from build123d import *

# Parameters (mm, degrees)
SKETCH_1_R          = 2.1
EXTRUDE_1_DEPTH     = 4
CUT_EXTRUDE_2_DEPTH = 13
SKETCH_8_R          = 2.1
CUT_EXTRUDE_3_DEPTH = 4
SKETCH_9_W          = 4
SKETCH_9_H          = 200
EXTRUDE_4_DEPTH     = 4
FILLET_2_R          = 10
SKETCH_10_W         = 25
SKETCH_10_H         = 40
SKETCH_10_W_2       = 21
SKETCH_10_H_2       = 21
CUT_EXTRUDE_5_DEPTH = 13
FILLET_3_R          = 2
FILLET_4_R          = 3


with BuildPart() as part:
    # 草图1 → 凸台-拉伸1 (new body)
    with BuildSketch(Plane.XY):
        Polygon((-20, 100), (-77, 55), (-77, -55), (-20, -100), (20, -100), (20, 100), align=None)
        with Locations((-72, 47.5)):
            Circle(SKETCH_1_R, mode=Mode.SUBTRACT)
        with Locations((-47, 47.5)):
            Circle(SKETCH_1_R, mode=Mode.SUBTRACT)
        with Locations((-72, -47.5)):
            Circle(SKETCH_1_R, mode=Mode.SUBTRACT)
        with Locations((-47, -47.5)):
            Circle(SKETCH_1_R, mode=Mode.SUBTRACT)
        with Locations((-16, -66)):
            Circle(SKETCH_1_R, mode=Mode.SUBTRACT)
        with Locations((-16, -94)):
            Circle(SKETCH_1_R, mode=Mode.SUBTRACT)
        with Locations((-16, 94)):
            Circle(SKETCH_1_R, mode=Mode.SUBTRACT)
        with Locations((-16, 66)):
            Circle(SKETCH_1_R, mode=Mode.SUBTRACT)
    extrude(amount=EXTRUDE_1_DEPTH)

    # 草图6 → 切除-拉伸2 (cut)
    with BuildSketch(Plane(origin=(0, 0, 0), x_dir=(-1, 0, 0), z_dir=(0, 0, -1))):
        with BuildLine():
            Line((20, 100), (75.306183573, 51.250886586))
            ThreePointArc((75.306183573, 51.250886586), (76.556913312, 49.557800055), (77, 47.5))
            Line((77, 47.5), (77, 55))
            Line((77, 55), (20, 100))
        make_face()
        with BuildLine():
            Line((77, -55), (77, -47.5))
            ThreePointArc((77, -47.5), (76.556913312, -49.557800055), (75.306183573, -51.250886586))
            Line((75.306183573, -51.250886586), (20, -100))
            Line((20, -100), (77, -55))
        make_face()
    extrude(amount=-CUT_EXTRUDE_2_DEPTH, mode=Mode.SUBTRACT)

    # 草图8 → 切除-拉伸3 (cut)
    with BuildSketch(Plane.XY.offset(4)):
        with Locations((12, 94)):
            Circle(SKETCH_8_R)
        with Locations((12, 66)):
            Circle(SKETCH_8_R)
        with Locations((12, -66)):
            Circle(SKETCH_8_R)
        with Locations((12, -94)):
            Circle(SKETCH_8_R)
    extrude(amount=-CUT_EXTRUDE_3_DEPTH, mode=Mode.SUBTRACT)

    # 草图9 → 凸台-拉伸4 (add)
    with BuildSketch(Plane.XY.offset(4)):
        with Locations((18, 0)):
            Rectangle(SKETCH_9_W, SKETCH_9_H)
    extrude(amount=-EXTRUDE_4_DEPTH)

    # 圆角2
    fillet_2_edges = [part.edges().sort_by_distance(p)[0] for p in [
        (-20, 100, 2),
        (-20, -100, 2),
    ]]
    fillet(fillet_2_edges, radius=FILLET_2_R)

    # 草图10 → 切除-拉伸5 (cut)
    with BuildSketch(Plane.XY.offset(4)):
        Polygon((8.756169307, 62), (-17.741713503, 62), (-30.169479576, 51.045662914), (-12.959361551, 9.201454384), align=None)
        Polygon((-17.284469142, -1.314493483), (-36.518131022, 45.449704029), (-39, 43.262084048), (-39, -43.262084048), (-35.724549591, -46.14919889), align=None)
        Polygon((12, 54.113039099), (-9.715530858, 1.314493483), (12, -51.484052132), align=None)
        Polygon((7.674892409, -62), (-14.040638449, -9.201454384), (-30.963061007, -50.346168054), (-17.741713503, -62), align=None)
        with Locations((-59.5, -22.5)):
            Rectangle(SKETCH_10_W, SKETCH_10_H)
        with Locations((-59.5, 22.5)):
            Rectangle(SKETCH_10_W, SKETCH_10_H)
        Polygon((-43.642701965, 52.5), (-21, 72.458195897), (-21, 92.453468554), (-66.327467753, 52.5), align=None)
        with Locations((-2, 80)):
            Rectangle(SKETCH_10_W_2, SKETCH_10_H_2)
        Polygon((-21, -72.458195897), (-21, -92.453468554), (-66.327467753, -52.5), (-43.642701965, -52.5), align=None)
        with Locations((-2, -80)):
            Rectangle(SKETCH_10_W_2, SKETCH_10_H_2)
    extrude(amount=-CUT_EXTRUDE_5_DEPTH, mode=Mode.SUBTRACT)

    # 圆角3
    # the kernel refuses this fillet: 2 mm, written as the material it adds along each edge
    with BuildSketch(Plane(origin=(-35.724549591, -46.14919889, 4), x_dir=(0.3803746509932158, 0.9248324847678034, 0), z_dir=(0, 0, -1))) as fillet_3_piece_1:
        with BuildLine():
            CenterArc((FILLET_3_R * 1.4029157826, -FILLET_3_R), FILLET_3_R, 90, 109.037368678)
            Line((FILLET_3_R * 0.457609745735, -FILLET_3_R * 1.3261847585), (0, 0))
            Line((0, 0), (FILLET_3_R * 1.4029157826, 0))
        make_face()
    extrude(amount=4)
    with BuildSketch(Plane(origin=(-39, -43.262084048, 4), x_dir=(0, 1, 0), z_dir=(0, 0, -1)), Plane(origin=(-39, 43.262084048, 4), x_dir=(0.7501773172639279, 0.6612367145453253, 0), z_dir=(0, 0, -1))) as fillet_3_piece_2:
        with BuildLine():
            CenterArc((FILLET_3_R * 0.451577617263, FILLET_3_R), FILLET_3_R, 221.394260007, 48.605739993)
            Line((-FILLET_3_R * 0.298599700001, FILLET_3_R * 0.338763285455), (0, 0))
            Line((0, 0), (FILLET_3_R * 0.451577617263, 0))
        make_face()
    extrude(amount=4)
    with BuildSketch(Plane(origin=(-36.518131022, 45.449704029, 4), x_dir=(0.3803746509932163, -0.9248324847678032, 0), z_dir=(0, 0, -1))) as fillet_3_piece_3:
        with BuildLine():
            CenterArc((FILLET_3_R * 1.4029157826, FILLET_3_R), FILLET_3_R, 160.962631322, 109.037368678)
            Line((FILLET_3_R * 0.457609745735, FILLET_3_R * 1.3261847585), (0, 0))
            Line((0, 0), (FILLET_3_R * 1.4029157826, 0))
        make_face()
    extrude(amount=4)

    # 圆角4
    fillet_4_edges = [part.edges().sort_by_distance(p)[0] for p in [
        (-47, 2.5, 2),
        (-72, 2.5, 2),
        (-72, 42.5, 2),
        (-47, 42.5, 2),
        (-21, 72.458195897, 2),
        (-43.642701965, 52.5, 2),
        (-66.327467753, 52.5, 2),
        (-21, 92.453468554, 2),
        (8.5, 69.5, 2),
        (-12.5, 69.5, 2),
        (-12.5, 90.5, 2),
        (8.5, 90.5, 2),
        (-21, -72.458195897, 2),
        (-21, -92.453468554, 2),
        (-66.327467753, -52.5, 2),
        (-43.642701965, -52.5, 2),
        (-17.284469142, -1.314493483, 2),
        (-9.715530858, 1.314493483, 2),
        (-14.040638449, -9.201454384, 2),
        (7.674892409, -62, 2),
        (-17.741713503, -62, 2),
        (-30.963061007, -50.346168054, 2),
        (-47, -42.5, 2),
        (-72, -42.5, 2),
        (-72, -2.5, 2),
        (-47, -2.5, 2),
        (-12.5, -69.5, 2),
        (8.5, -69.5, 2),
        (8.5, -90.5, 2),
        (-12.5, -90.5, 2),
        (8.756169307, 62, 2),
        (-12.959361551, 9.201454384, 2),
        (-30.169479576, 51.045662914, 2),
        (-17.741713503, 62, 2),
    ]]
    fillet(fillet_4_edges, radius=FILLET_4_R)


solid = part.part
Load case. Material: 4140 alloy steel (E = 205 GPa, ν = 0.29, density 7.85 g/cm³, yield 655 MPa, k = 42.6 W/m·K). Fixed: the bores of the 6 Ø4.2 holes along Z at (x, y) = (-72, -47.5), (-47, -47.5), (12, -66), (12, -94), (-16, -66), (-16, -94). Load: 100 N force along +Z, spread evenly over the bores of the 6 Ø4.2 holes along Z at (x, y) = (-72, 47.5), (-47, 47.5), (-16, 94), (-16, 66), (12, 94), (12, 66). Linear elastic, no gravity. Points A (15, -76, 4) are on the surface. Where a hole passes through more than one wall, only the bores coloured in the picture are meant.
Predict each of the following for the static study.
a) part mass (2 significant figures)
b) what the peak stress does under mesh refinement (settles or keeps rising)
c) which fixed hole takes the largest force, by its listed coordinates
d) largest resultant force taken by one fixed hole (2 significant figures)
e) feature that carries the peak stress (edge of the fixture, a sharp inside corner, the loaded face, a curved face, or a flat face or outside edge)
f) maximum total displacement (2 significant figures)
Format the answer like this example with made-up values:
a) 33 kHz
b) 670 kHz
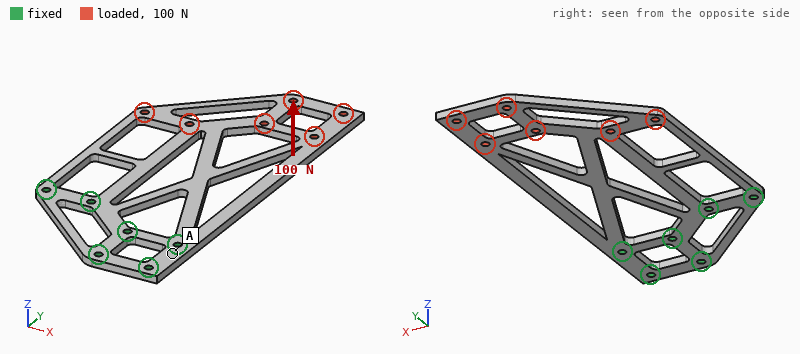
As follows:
a) 250 g
b) keeps rising
c) (-47, -47.5)
d) 120 N
e) edge of the fixture
f) 2.5 mm
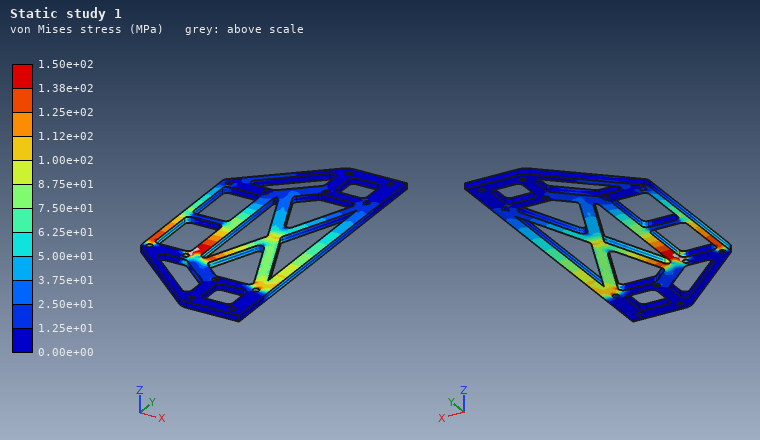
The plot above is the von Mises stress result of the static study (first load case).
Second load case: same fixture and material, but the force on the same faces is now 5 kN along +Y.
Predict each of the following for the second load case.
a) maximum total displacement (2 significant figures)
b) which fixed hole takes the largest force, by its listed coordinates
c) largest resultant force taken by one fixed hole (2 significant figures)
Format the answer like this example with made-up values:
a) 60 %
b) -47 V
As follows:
a) 57 µm
b) (12, -66)
c) 2.2 kN
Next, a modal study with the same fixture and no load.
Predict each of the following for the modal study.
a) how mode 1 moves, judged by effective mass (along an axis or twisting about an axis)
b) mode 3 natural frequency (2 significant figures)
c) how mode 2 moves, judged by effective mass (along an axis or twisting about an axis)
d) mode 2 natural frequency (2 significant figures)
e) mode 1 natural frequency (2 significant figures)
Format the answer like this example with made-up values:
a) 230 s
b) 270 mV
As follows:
a) along Z
b) 780 Hz
c) twisting about Y
d) 450 Hz
e) 130 Hz
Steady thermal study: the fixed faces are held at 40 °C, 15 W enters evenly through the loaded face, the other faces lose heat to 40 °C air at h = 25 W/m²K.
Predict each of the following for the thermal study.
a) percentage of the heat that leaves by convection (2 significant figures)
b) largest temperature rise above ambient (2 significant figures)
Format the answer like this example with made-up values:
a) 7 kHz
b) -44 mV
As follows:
a) 92 %
b) 74 K
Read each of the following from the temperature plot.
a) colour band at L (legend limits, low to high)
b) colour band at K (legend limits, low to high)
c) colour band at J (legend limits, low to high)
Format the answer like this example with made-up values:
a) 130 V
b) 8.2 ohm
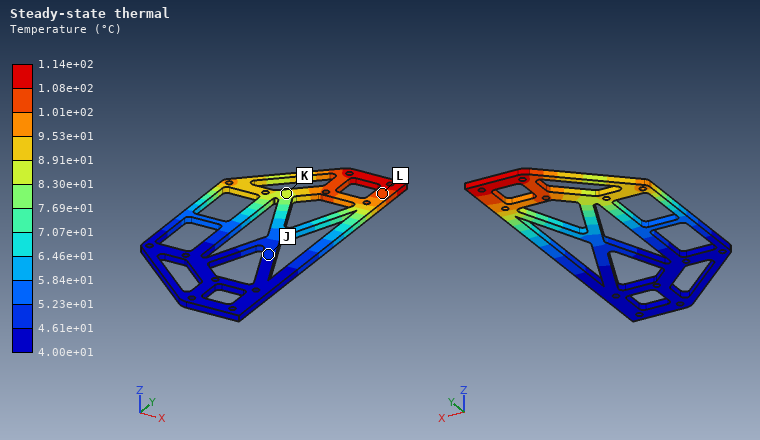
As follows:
a) 1.01e+02 to 1.08e+02 °C
b) 8.30e+01 to 8.91e+01 °C
c) 4.61e+01 to 5.23e+01 °C
